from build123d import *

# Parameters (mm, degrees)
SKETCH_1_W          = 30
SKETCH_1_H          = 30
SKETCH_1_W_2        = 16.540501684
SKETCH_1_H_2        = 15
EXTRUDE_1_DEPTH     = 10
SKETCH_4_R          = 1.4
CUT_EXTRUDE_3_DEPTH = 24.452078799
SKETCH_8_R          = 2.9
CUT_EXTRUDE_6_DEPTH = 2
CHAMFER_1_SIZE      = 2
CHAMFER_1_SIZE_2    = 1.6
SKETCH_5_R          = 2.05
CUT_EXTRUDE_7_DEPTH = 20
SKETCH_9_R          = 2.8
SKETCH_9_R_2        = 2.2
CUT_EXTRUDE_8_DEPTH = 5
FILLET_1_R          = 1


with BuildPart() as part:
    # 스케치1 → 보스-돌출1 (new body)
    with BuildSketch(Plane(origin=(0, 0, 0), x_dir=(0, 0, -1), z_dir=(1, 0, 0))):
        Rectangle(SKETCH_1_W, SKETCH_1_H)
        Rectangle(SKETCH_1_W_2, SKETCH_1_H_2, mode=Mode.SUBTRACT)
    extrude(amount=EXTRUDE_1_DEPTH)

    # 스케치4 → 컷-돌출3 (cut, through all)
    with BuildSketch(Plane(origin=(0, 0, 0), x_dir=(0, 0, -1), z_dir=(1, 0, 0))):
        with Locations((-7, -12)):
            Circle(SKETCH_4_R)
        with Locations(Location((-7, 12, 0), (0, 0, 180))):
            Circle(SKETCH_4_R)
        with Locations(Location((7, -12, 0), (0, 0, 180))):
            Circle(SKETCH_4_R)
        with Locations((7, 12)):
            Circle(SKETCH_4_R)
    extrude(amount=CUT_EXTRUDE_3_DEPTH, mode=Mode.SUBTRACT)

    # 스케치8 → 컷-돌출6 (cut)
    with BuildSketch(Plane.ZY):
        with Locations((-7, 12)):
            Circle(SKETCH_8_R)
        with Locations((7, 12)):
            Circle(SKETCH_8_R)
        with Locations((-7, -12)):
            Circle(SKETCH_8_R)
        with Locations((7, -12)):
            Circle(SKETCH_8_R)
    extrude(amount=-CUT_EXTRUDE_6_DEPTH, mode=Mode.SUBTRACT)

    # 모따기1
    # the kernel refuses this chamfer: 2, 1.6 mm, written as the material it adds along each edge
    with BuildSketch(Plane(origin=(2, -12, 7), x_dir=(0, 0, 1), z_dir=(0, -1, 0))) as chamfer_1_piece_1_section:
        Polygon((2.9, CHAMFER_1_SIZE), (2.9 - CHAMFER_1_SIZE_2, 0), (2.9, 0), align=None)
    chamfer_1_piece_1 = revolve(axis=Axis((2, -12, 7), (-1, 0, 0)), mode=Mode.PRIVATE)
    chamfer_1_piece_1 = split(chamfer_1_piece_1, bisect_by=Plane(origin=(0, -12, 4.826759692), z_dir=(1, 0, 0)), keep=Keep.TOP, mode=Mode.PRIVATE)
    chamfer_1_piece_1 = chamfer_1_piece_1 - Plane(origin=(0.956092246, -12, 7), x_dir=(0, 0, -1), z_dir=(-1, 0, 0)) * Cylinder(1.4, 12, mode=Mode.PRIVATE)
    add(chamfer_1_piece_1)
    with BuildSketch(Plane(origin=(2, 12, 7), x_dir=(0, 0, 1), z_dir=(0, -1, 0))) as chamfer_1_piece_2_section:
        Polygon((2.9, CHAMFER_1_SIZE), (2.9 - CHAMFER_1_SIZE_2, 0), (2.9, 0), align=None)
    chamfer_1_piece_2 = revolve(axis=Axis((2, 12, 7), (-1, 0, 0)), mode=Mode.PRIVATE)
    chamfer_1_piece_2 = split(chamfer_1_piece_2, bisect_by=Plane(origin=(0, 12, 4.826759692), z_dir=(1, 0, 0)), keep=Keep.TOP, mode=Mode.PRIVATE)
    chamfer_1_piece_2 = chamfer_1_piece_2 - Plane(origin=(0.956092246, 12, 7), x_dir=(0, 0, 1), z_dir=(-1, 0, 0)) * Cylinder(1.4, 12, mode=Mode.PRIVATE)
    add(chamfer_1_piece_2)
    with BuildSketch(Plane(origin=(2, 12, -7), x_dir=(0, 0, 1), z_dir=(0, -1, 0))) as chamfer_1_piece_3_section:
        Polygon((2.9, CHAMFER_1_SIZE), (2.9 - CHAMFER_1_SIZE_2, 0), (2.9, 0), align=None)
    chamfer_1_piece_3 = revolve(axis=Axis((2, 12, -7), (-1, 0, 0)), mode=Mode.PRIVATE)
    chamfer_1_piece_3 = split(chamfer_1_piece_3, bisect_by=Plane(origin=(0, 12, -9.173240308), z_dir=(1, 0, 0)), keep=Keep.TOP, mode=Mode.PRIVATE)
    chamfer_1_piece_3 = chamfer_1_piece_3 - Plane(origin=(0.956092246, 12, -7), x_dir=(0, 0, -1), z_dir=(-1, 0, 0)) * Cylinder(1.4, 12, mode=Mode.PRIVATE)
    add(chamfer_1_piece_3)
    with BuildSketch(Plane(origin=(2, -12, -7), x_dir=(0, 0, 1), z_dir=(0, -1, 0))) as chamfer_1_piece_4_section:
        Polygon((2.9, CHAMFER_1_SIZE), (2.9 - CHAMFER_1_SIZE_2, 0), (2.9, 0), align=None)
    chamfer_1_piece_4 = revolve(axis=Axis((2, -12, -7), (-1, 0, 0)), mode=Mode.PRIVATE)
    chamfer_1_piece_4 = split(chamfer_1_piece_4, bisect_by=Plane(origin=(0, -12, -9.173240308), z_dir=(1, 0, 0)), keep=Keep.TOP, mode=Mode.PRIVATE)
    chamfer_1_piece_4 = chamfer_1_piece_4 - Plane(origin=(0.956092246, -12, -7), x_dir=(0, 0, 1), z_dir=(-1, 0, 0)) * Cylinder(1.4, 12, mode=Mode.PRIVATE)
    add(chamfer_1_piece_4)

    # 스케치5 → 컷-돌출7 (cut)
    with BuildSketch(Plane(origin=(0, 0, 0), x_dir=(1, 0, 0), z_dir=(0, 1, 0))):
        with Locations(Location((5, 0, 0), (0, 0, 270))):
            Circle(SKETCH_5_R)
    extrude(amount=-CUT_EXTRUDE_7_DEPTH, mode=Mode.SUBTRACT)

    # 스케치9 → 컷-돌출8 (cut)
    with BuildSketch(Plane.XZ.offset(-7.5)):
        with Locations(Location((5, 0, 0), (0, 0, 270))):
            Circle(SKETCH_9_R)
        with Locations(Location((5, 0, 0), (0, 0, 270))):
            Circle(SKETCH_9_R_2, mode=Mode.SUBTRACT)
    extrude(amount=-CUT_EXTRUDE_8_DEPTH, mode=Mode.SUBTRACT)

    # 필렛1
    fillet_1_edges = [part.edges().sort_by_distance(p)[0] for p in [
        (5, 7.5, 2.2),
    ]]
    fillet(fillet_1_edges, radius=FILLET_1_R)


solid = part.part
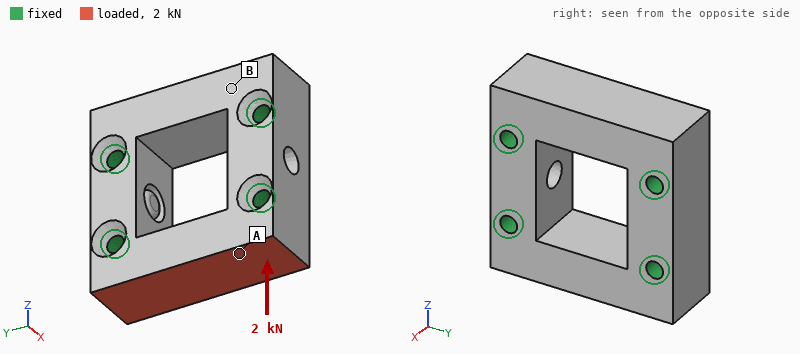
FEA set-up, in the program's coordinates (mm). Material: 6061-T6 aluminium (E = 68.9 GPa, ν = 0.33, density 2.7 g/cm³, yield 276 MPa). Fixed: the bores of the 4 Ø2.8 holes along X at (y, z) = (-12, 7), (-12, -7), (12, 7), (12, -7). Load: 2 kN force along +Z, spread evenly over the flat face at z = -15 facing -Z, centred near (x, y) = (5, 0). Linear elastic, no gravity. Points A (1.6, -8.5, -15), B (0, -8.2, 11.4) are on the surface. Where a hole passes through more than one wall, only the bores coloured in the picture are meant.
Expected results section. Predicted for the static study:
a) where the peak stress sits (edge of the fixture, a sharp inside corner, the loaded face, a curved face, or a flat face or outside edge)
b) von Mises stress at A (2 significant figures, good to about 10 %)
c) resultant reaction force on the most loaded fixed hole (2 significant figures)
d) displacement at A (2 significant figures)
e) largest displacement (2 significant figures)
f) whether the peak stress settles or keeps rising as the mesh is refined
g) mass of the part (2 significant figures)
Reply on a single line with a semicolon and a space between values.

edge of the fixture; 7.7 MPa; 1000 N; 2.8 µm; 5.5 µm; keeps rising; 16 g
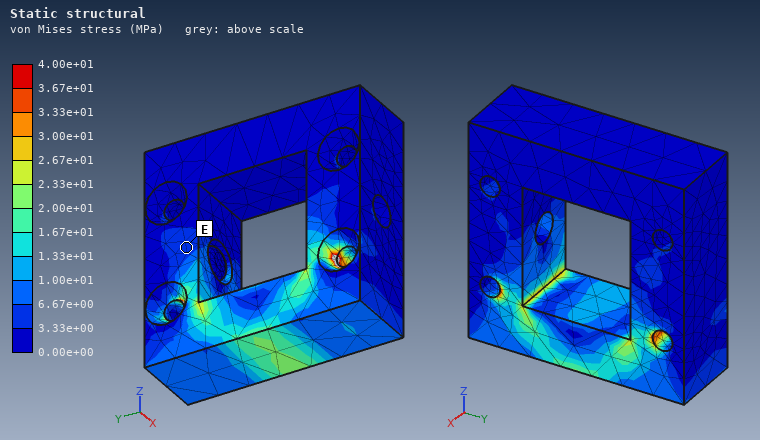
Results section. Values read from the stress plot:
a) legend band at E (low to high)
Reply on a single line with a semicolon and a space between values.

3.33e+00 to 6.67e+00 MPa
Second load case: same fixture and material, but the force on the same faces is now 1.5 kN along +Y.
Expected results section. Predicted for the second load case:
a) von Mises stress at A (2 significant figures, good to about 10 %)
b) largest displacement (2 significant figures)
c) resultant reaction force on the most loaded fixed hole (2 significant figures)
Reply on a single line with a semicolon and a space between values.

13 MPa; 4.6 µm; 870 N
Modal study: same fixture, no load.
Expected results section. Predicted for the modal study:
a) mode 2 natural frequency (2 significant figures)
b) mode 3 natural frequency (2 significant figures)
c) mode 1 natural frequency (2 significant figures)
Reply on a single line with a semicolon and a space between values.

38 kHz; 47 kHz; 38 kHz
